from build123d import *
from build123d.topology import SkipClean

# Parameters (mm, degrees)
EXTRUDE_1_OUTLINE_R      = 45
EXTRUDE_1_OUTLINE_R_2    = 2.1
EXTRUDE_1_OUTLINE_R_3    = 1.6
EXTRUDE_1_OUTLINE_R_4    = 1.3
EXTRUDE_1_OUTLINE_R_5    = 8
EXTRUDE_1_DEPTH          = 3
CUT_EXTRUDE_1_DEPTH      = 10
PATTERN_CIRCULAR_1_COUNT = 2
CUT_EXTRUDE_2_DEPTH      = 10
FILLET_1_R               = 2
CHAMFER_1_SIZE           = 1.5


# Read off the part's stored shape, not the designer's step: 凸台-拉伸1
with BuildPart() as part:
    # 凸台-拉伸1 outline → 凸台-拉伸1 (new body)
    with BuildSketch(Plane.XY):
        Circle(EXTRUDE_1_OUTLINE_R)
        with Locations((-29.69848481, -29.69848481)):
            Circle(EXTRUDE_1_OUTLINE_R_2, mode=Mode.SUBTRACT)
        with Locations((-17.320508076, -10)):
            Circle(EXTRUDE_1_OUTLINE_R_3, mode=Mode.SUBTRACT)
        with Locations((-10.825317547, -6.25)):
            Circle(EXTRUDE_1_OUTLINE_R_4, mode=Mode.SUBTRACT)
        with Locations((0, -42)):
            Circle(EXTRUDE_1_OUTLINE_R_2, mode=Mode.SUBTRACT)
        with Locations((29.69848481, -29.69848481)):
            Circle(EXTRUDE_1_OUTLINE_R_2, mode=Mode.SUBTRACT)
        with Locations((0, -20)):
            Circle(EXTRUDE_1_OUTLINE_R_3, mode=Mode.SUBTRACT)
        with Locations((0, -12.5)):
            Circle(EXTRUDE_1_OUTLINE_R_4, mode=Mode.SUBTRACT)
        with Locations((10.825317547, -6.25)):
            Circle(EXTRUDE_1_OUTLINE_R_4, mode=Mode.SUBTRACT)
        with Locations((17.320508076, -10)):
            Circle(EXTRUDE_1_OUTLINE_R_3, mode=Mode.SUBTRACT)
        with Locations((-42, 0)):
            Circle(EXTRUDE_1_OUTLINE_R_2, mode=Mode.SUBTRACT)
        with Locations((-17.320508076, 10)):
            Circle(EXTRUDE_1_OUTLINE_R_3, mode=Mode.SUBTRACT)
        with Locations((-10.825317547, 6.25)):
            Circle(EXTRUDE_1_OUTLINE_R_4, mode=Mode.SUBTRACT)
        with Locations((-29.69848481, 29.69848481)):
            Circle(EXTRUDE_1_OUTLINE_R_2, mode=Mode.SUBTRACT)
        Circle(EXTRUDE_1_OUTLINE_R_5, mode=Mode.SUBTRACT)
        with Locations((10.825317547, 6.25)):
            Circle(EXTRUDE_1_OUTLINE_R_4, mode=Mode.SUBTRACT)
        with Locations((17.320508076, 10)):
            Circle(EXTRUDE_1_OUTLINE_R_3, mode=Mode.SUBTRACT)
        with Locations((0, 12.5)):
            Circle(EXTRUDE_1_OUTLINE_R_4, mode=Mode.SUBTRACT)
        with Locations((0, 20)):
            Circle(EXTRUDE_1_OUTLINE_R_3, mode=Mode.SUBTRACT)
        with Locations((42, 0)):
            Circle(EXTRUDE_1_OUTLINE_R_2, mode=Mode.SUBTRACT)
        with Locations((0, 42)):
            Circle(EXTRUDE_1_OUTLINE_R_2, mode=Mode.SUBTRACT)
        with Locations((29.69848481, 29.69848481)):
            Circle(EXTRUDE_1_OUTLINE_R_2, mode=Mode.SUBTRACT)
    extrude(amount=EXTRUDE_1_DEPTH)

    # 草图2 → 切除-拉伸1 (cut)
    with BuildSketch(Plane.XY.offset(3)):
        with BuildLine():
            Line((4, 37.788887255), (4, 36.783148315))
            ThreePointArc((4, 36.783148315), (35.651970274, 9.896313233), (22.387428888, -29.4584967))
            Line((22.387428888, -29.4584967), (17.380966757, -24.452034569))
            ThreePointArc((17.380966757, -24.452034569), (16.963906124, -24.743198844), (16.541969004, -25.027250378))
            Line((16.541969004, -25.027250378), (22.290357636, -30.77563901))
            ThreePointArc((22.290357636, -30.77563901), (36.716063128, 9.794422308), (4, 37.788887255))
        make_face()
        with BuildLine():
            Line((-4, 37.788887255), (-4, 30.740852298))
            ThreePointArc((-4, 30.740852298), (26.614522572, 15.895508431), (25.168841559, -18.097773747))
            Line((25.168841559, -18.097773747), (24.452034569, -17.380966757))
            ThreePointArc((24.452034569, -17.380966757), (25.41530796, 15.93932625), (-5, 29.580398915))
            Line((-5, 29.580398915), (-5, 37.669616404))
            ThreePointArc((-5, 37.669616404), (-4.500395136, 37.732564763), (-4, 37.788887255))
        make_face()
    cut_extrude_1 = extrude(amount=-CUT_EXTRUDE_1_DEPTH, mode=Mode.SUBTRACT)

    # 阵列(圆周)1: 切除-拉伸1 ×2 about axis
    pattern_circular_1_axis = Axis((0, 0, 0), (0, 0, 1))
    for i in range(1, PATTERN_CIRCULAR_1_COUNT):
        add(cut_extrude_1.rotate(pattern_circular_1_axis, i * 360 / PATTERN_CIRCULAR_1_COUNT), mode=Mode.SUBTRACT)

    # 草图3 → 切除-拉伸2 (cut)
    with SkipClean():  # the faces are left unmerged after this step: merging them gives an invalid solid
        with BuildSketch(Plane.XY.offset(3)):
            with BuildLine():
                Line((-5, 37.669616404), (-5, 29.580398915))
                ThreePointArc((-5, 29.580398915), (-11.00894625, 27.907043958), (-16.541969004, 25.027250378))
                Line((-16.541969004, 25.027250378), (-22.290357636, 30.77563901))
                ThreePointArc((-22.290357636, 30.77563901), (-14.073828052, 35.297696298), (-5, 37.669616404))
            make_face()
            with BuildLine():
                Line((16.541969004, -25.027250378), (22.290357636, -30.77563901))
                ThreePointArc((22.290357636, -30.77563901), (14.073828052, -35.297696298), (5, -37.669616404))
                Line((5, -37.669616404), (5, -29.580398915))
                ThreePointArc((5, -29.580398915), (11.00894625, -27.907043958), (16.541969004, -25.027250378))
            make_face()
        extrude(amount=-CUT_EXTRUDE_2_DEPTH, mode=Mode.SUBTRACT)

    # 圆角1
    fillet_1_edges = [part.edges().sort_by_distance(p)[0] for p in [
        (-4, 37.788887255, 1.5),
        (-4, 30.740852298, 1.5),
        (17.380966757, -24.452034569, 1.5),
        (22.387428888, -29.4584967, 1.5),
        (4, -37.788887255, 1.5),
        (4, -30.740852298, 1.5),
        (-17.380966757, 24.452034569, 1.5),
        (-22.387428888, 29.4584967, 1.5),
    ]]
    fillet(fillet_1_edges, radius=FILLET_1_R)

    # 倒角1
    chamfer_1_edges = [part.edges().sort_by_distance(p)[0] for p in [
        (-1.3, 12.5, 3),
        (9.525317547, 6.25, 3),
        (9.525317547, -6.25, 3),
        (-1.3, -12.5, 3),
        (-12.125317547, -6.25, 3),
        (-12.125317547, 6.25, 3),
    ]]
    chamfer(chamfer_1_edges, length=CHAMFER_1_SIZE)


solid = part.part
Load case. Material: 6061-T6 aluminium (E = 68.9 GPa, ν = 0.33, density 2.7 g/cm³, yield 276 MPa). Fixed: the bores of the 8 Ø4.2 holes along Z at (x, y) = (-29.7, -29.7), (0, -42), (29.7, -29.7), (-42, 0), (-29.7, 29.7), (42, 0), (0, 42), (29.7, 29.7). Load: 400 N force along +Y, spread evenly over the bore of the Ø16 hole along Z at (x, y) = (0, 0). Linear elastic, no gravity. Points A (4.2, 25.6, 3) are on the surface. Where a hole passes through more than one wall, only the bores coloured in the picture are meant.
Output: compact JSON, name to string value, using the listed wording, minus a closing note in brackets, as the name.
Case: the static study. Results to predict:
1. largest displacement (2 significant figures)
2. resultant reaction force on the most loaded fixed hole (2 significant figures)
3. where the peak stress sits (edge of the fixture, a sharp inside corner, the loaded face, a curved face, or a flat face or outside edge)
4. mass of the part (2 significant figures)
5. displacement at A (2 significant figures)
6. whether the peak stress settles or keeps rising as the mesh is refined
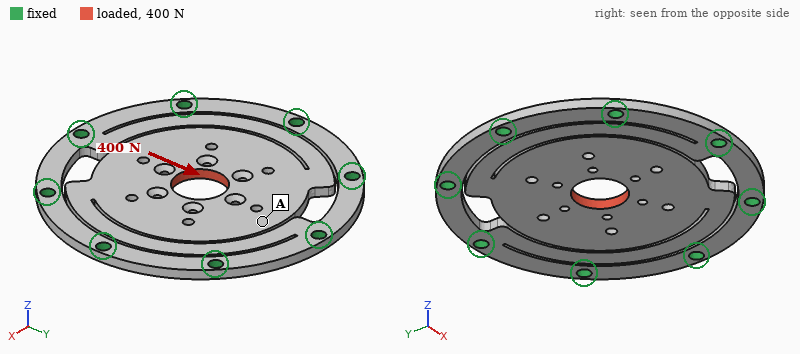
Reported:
{"largest displacement": "0.75 mm", "resultant reaction force on the most loaded fixed hole": "230 N", "where the peak stress sits": "a sharp inside corner", "mass of the part": "43 g", "displacement at A": "0.75 mm", "whether the peak stress settles or keeps rising as the mesh is refined": "keeps rising"}
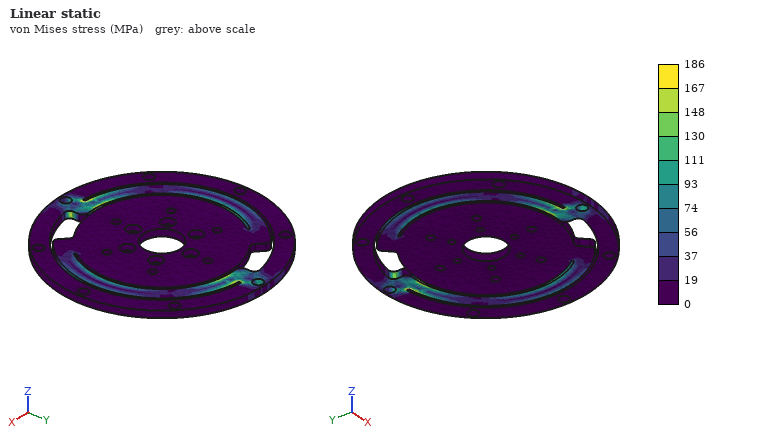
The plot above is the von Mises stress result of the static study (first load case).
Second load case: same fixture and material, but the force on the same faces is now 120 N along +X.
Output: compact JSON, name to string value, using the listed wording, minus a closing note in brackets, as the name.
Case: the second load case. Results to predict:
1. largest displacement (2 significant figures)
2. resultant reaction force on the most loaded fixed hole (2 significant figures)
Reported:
{"largest displacement": "0.50 mm", "resultant reaction force on the most loaded fixed hole": "84 N"}
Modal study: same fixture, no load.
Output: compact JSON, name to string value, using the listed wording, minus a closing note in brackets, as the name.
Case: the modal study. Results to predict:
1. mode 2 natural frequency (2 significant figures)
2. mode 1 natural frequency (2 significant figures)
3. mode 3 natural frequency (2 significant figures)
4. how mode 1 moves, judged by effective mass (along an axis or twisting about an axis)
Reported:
{"mode 2 natural frequency": "270 Hz", "mode 1 natural frequency": "220 Hz", "mode 3 natural frequency": "480 Hz", "how mode 1 moves, judged by effective mass": "along Z"}
